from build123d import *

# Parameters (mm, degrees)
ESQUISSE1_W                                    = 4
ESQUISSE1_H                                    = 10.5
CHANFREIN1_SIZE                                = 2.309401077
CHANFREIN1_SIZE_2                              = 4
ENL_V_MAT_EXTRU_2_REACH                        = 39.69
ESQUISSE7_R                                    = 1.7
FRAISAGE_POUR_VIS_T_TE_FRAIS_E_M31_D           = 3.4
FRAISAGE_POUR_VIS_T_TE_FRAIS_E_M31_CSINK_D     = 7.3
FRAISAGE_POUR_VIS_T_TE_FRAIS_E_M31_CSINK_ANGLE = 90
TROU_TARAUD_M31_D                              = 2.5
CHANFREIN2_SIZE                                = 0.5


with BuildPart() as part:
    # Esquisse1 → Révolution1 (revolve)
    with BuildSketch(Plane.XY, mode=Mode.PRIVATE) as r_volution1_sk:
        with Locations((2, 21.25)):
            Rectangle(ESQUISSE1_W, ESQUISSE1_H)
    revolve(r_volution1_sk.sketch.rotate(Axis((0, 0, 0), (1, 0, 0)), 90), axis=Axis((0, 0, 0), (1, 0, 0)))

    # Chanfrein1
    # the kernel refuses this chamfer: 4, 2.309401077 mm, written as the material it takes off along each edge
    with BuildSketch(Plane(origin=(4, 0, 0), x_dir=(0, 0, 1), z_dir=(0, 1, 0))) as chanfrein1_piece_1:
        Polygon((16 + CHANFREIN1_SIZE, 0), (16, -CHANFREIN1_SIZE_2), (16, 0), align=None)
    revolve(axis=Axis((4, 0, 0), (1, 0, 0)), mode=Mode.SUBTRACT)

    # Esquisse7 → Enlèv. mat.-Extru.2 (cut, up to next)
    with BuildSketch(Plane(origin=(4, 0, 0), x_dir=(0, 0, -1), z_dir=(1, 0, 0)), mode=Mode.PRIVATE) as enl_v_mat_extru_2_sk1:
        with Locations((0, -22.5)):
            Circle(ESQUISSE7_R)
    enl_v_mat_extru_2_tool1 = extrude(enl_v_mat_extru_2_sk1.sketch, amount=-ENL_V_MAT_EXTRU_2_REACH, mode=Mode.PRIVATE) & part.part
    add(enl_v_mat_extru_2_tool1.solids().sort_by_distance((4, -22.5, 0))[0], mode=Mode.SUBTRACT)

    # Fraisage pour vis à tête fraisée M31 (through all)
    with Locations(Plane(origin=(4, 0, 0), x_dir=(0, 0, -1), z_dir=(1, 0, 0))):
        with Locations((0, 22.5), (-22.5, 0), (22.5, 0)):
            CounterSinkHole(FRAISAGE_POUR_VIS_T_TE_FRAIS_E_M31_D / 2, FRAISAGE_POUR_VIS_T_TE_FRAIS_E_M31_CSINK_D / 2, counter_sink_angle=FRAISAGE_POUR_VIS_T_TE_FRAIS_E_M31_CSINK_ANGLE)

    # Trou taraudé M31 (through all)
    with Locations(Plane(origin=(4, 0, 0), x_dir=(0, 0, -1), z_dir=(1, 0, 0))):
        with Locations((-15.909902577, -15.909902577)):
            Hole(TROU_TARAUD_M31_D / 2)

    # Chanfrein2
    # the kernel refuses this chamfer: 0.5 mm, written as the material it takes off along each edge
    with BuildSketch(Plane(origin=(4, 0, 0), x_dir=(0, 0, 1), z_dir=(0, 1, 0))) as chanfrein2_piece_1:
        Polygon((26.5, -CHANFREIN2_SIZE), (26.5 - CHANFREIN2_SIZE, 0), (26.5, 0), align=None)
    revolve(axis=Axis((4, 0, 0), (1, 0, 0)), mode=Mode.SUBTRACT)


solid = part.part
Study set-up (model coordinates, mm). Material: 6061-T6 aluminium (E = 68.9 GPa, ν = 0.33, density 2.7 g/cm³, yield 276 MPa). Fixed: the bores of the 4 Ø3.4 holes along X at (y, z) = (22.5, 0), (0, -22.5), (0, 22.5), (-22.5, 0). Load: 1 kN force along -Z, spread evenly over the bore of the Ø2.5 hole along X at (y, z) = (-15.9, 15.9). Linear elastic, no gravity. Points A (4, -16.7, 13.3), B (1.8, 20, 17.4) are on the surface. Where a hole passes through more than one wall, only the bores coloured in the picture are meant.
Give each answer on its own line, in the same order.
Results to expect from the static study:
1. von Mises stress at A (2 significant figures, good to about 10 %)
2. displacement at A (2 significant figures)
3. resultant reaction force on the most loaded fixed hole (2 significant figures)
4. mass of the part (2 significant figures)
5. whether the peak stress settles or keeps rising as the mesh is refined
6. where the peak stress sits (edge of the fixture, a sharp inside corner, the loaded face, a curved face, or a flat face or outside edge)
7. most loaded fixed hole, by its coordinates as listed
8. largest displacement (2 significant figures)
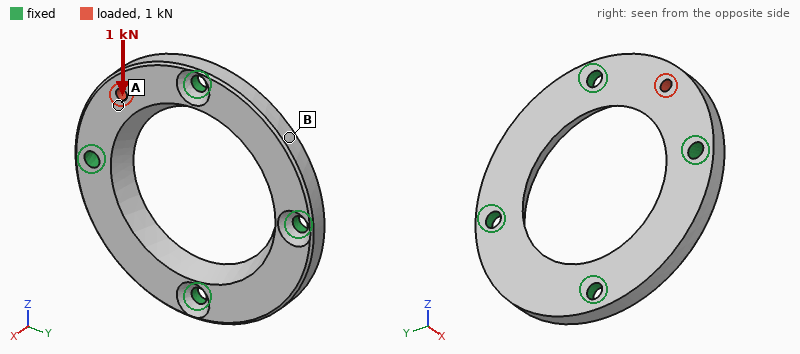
36 MPa
9.6 µm
880 N
13 g
keeps rising
edge of the fixture
(-22.5, 0)
12 µm
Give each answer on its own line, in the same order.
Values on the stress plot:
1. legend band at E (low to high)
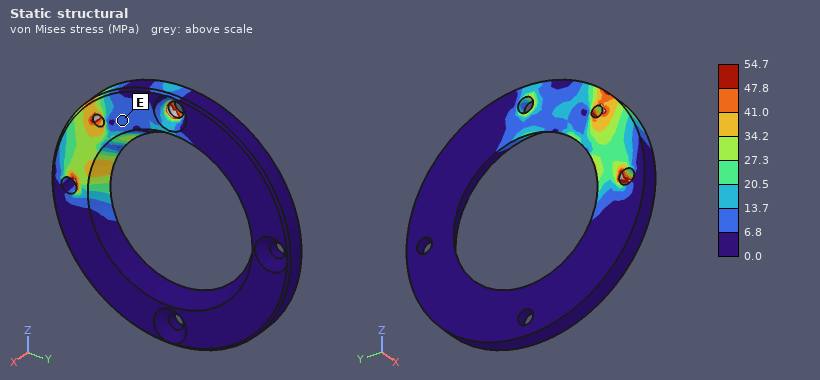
6.8 to 13.7 MPa
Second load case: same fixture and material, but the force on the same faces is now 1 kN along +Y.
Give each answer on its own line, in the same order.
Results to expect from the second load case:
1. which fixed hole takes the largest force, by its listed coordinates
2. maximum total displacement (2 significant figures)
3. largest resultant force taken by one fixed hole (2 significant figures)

(0, 22.5)
13 µm
840 N
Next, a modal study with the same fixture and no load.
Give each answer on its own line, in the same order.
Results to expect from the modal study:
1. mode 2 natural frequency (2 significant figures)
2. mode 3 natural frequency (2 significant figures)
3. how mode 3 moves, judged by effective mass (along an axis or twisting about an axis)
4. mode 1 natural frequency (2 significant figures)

13 kHz
14 kHz
twisting about Y
12 kHz
